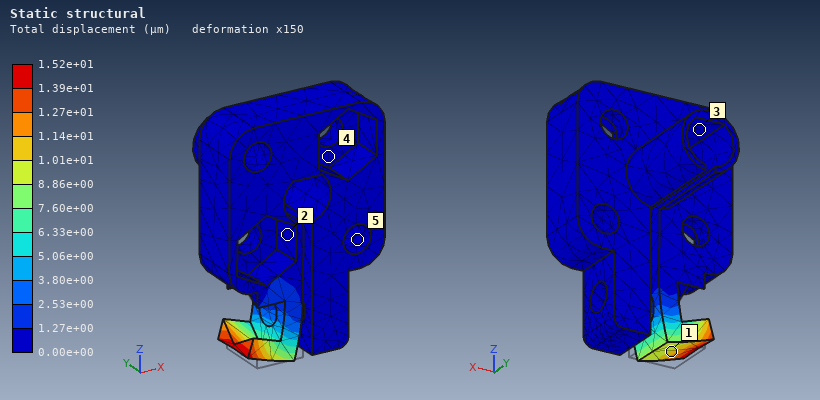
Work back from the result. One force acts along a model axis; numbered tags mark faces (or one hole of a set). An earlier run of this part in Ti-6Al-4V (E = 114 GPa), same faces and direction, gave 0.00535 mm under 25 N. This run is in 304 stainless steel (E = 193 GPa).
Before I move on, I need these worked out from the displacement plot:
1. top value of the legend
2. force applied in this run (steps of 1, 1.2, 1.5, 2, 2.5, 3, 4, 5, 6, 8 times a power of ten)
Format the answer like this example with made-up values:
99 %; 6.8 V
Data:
1.52e+01 µm; 120 N
